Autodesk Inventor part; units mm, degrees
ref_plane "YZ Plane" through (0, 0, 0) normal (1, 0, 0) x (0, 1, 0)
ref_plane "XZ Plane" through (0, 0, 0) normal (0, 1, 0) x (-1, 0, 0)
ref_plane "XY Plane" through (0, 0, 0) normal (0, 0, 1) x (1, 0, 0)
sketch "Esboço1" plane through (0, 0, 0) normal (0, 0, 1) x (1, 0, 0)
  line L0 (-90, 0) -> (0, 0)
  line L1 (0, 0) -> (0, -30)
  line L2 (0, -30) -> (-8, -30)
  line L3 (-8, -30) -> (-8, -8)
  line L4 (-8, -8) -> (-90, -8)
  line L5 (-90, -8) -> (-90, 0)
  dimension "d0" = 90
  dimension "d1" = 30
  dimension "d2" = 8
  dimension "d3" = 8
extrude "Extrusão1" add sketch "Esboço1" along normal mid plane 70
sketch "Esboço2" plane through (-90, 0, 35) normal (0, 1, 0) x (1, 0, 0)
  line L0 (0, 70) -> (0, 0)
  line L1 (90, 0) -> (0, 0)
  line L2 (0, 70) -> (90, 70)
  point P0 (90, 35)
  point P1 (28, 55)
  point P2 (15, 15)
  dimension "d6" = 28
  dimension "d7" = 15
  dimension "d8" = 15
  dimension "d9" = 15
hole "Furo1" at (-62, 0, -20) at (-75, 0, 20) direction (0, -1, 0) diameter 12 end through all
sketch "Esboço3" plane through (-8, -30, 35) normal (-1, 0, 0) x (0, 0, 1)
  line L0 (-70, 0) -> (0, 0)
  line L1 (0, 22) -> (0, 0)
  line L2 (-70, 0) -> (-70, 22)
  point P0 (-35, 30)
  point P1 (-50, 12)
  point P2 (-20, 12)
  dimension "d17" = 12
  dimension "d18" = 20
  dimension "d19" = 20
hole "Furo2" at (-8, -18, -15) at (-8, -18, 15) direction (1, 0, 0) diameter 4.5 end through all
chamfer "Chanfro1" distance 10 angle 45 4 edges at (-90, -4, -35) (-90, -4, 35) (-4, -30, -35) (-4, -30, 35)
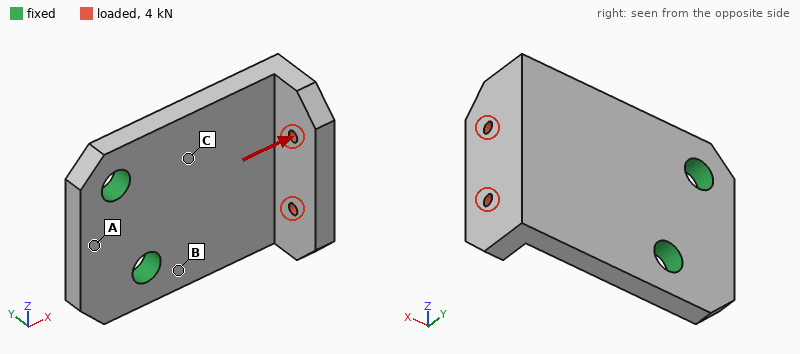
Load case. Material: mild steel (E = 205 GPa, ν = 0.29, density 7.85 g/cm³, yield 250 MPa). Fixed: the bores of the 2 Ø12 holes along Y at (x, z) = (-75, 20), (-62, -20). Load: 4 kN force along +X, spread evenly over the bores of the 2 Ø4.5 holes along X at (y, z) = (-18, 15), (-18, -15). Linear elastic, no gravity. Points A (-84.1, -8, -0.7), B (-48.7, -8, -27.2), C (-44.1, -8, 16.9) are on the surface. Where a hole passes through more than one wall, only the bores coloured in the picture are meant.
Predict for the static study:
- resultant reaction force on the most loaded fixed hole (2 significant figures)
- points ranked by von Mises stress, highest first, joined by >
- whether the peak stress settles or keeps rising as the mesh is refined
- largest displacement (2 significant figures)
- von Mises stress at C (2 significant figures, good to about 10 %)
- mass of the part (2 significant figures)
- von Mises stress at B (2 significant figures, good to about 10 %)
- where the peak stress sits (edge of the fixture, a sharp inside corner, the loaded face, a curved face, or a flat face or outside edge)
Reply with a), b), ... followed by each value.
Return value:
a) 2.1 kN
b) B > C > A
c) keeps rising
d) 0.23 mm
e) 70 MPa
f) 460 g
g) 90 MPa
h) edge of the fixture
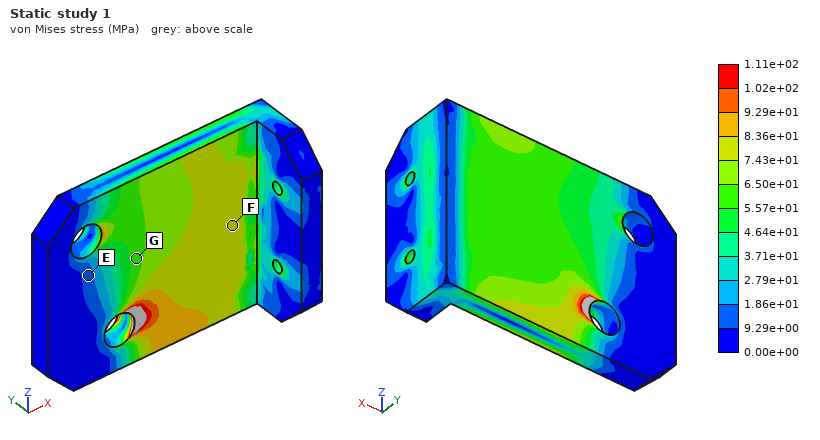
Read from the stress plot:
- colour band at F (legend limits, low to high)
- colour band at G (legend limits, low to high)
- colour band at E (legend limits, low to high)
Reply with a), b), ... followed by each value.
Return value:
a) 7.43e+01 to 8.36e+01 MPa
b) 5.57e+01 to 6.50e+01 MPa
c) 9.29e+00 to 1.86e+01 MPa
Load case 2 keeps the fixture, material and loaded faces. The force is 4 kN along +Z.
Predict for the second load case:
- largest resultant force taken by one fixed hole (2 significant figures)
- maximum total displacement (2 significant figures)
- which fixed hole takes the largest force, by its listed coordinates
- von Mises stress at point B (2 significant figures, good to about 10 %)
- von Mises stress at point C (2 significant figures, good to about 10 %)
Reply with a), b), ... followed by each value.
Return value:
a) 6.0 kN
b) 0.12 mm
c) (-62, -20)
d) 50 MPa
e) 57 MPa
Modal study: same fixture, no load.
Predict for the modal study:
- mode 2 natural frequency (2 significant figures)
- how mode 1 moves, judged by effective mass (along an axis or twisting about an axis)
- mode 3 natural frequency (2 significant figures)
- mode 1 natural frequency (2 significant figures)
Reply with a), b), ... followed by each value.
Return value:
a) 2400 Hz
b) along Y
c) 5100 Hz
d) 1100 Hz
